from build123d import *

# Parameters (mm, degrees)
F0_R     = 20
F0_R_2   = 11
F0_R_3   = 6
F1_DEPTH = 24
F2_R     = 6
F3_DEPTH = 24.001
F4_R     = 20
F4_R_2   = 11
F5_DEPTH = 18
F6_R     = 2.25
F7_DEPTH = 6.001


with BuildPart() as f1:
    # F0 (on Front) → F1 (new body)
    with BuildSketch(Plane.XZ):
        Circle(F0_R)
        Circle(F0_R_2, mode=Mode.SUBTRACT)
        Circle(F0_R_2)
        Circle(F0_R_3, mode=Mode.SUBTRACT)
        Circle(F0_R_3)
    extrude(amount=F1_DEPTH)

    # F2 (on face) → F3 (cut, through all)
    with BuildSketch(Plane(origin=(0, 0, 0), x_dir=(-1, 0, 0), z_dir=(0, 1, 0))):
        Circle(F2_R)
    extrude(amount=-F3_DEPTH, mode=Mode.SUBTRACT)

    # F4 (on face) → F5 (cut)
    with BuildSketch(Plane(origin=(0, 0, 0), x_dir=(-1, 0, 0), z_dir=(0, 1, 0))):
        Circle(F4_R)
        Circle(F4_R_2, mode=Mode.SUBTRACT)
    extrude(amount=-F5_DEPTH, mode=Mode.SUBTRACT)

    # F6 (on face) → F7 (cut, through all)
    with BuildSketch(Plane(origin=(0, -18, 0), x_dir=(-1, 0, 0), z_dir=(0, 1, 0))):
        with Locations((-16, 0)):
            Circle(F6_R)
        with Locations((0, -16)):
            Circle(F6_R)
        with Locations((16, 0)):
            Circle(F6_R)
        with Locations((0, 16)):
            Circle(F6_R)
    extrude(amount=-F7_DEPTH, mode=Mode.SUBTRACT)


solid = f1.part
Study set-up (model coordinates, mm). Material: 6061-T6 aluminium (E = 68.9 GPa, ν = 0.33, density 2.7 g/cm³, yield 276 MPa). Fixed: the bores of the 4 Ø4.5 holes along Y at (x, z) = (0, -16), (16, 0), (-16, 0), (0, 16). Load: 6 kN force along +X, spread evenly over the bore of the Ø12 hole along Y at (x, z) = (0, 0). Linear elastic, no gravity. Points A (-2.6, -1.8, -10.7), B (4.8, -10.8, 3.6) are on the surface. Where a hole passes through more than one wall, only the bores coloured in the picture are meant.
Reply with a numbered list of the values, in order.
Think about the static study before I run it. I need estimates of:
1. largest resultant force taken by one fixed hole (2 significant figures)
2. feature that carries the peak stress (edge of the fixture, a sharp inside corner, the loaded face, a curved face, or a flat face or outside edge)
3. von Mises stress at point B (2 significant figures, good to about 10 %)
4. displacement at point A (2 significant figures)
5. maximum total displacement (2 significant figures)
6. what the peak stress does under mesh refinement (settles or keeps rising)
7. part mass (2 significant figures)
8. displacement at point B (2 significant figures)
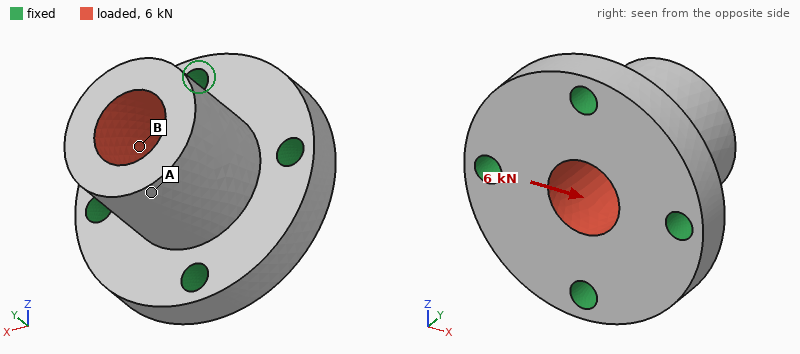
1. 2.6 kN
2. edge of the fixture
3. 30 MPa
4. 26 µm
5. 32 µm
6. keeps rising
7. 30 g
8. 16 µm
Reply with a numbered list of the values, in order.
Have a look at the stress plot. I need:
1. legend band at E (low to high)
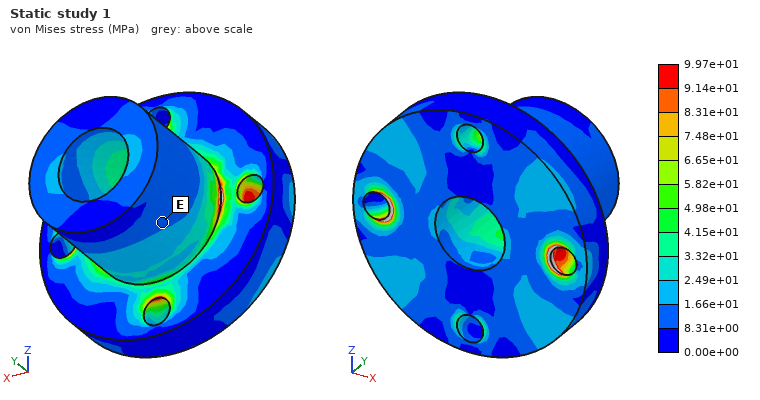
1. 8.31e+00 to 1.66e+01 MPa
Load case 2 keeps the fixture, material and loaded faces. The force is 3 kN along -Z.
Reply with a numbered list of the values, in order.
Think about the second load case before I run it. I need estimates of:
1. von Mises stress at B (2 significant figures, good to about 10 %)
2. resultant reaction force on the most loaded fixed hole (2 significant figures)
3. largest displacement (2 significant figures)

1. 18 MPa
2. 1.3 kN
3. 16 µm
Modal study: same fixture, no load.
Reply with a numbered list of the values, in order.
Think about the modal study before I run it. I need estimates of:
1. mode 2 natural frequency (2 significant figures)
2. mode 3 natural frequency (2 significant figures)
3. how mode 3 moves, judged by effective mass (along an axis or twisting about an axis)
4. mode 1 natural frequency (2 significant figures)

1. 19 kHz
2. 30 kHz
3. along Y
4. 19 kHz
